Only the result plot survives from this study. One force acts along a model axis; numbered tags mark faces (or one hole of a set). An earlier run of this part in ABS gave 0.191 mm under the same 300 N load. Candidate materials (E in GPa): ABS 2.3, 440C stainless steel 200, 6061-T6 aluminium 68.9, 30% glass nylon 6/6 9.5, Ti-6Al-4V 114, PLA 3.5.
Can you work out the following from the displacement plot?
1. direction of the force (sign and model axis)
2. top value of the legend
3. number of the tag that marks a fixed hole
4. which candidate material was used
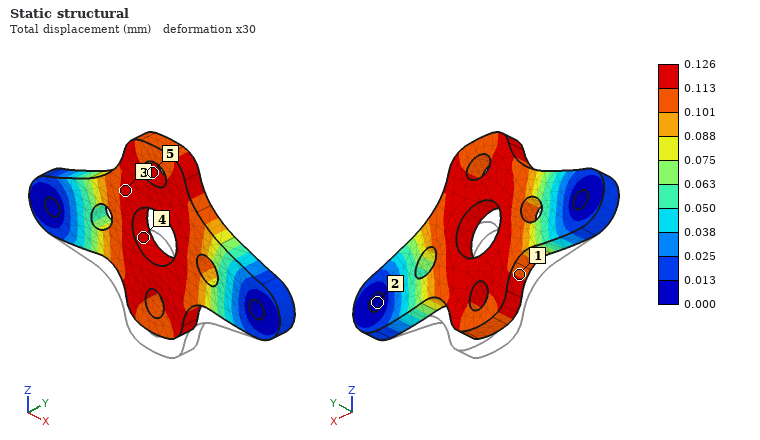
+Z
0.126 mm
2
PLA
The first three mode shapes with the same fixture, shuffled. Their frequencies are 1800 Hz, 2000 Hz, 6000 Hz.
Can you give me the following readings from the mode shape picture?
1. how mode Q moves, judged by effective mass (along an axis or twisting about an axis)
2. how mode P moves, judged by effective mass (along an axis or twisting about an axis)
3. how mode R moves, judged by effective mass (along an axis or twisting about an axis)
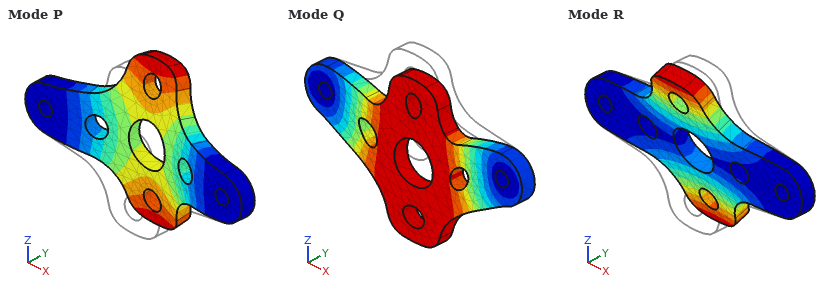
along Z
along Y
twisting about X
